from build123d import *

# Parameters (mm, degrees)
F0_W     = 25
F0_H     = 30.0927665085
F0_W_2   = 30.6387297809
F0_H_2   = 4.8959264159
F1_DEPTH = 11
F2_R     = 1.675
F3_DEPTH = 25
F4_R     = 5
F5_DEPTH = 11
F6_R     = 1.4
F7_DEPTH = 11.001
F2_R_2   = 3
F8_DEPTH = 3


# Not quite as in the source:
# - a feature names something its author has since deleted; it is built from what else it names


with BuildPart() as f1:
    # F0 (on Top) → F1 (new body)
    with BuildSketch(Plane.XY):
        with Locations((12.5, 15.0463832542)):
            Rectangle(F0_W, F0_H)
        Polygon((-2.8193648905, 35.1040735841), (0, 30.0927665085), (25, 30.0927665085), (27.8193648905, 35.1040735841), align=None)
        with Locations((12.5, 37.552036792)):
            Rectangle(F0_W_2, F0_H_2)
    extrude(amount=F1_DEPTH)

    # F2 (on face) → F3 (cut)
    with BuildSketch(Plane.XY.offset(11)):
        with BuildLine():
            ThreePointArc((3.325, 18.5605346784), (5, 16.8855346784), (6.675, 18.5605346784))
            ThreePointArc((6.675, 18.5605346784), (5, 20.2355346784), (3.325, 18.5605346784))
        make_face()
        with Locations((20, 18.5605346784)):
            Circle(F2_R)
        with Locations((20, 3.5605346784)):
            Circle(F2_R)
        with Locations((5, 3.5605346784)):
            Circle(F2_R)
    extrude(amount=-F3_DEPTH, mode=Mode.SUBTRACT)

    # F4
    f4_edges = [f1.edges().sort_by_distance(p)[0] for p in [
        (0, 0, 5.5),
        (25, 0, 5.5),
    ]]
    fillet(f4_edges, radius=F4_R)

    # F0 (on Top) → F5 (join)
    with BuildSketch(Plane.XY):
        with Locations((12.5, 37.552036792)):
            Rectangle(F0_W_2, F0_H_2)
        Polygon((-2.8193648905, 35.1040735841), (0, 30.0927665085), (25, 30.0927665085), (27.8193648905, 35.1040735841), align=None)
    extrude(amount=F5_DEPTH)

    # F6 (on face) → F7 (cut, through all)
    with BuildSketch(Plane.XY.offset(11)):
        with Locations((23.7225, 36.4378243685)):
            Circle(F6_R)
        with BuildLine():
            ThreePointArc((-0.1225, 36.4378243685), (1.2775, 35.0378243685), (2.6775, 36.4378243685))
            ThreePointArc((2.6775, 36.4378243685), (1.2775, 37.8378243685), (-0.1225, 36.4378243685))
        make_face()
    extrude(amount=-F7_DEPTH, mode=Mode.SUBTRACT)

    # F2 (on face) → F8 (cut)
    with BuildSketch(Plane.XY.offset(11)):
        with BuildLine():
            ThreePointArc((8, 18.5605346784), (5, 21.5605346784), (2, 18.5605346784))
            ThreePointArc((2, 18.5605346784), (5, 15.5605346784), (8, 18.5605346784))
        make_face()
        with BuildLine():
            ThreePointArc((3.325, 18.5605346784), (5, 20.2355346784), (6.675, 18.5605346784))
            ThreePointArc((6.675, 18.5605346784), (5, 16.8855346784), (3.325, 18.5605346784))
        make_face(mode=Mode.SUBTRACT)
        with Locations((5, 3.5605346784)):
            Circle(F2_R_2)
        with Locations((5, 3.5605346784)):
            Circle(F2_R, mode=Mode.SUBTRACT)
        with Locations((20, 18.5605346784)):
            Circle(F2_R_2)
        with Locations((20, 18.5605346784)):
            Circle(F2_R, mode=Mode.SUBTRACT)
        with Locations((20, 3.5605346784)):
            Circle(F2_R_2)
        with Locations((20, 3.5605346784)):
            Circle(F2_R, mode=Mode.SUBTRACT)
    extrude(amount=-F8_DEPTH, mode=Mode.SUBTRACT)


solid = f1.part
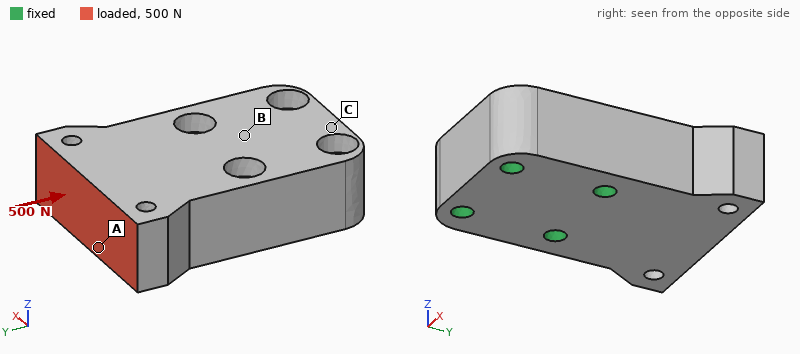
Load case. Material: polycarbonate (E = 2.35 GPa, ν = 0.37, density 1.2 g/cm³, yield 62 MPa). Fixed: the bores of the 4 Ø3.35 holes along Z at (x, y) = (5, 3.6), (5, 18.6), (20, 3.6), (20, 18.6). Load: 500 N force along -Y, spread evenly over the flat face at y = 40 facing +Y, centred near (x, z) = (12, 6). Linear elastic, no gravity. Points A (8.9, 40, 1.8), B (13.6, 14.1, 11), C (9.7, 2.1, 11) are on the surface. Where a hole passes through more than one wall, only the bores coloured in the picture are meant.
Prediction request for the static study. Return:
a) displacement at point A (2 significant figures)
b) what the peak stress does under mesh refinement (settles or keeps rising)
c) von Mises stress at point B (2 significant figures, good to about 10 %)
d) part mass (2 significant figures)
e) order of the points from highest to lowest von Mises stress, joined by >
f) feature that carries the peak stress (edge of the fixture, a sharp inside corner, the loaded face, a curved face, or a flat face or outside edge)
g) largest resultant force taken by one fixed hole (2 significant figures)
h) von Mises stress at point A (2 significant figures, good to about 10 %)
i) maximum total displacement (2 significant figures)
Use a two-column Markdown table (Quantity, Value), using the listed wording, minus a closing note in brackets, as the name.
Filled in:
| Quantity | Value |
|---|---|
| displacement at point A | 20 µm |
| what the peak stress does under mesh refinement | keeps rising |
| von Mises stress at point B | 1.1 MPa |
| part mass | 13 g |
| order of the points from highest to lowest von Mises stress, joined by > | A > B > C |
| feature that carries the peak stress | edge of the fixture |
| largest resultant force taken by one fixed hole | 210 N |
| von Mises stress at point A | 2.0 MPa |
| maximum total displacement | 32 µm |
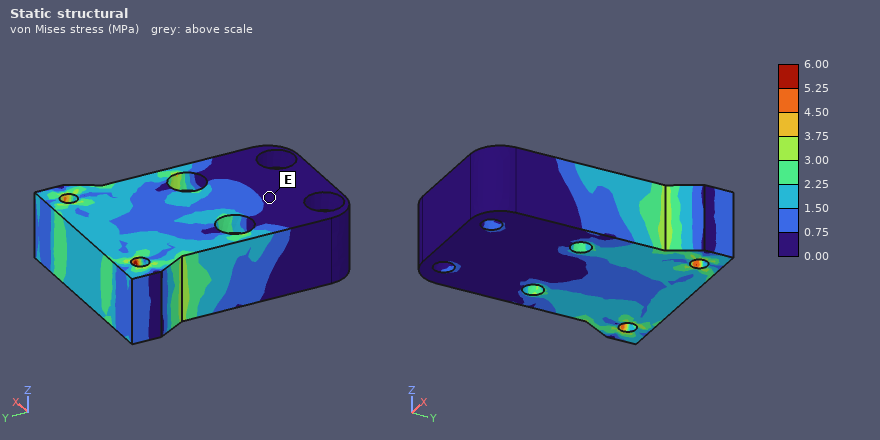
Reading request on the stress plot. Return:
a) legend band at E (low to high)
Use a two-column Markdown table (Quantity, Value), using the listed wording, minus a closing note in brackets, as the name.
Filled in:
| Quantity | Value |
|---|---|
| legend band at E | 0.00 to 0.75 MPa |
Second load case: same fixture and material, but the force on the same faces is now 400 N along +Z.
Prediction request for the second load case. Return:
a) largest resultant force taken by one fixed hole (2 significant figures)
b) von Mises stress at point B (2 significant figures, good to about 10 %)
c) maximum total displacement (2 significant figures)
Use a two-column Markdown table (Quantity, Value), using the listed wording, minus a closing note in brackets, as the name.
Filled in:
| Quantity | Value |
|---|---|
| largest resultant force taken by one fixed hole | 310 N |
| von Mises stress at point B | 7.8 MPa |
| maximum total displacement | 0.35 mm |
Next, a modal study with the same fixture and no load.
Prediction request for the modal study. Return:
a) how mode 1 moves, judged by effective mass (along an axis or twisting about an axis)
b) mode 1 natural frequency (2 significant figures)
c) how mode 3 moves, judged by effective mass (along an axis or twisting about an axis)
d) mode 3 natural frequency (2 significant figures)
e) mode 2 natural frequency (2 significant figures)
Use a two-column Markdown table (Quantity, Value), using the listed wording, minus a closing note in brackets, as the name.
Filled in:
| Quantity | Value |
|---|---|
| how mode 1 moves, judged by effective mass | along Z |
| mode 1 natural frequency | 3600 Hz |
| how mode 3 moves, judged by effective mass | along X |
| mode 3 natural frequency | 6200 Hz |
| mode 2 natural frequency | 6000 Hz |
